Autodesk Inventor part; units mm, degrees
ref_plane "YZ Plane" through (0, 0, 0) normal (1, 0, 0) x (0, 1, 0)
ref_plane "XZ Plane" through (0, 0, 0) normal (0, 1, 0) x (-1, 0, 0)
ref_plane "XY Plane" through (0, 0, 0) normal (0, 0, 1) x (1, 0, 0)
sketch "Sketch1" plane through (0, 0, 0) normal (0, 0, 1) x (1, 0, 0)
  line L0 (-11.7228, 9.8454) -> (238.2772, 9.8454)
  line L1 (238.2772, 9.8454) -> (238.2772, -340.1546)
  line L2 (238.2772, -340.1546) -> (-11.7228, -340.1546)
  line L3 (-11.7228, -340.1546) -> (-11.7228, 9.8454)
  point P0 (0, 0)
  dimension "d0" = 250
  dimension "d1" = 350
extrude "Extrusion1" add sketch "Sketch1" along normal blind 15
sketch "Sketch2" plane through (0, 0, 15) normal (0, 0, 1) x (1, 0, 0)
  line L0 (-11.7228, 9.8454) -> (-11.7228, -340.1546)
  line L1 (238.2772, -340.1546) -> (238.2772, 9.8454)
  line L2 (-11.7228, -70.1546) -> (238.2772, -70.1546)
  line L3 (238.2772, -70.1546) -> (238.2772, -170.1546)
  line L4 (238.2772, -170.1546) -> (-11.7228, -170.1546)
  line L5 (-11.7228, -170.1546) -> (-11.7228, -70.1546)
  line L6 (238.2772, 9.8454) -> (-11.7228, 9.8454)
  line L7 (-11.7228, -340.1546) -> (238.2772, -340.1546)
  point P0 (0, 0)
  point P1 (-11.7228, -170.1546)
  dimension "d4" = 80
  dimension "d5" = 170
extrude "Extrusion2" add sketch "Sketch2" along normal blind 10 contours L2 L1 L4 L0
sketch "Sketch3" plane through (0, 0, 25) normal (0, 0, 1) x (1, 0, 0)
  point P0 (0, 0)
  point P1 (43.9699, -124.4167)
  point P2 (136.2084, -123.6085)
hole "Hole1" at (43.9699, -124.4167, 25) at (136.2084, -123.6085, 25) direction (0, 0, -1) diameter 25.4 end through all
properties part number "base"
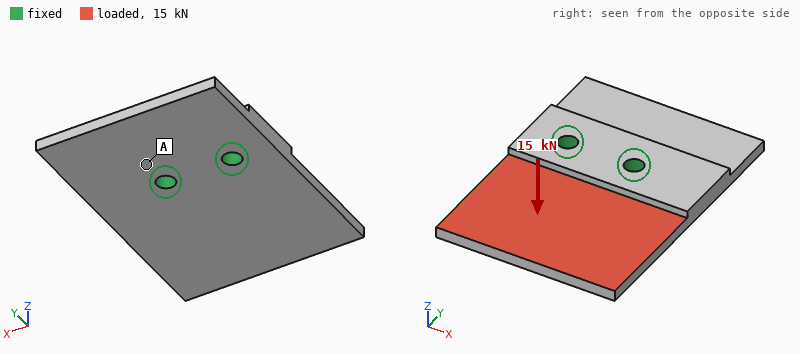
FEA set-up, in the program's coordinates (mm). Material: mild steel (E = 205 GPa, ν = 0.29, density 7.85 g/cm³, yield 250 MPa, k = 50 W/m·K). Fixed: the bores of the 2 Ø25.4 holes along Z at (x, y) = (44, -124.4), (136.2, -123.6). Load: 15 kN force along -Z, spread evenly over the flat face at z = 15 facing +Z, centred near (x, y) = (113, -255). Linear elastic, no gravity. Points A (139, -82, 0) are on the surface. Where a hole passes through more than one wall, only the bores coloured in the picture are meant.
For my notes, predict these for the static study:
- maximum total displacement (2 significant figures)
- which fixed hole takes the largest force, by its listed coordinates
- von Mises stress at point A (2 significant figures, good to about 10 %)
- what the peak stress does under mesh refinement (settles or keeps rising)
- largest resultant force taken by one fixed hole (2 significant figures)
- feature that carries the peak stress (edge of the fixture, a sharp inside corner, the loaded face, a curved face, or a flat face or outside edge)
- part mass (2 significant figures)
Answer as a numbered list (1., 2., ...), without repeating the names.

1. 0.94 mm
2. (136.2, -123.6)
3. 13 MPa
4. keeps rising
5. 9.5 kN
6. edge of the fixture
7. 12 kg
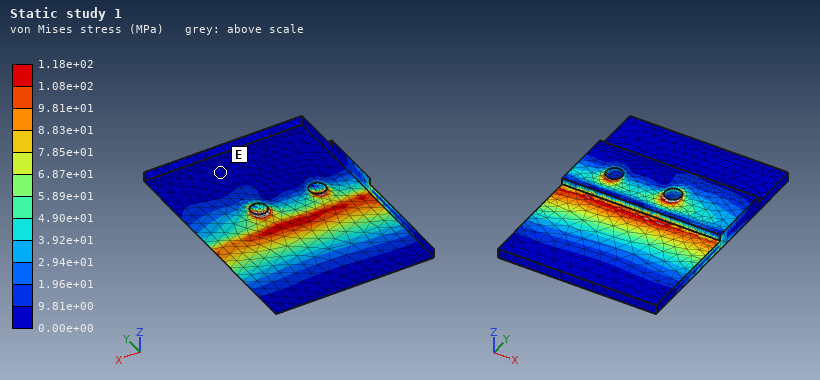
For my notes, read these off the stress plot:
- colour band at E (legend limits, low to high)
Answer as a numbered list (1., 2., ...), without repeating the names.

1. 0.00e+00 to 9.81e+00 MPa
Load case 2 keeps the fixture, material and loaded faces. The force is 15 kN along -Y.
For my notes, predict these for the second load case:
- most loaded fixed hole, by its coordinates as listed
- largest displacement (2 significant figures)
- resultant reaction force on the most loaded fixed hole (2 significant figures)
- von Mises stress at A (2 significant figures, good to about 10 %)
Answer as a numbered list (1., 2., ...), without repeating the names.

1. (136.2, -123.6)
2. 84 µm
3. 11 kN
4. 2.5 MPa
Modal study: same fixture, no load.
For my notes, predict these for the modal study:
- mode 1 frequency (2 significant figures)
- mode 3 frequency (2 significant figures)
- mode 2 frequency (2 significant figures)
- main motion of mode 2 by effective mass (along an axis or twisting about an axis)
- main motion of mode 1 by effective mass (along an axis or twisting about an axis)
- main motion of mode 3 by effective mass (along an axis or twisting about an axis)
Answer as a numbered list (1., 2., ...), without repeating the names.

1. 360 Hz
2. 1100 Hz
3. 660 Hz
4. twisting about Y
5. along Z
6. along Z
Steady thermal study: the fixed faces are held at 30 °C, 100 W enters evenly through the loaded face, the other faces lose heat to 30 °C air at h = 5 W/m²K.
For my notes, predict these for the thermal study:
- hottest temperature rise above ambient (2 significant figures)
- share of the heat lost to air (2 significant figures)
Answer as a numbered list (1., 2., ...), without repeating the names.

1. 57 K
2. 14 %
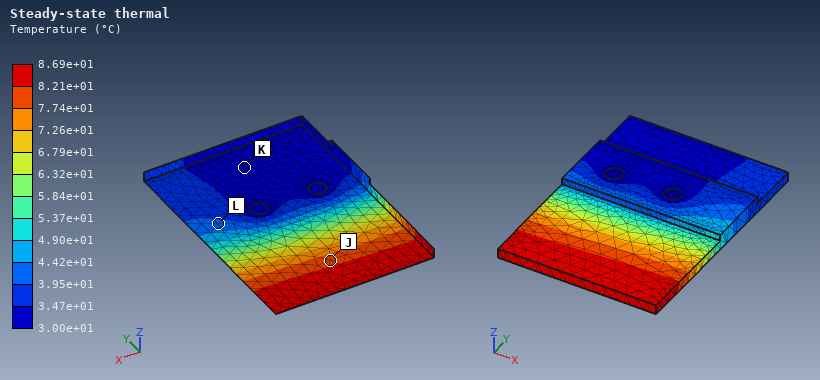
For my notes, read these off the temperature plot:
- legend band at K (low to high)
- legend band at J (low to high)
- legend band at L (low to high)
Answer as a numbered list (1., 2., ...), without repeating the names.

1. 3.00e+01 to 3.47e+01 °C
2. 7.74e+01 to 8.21e+01 °C
3. 3.95e+01 to 4.42e+01 °C
